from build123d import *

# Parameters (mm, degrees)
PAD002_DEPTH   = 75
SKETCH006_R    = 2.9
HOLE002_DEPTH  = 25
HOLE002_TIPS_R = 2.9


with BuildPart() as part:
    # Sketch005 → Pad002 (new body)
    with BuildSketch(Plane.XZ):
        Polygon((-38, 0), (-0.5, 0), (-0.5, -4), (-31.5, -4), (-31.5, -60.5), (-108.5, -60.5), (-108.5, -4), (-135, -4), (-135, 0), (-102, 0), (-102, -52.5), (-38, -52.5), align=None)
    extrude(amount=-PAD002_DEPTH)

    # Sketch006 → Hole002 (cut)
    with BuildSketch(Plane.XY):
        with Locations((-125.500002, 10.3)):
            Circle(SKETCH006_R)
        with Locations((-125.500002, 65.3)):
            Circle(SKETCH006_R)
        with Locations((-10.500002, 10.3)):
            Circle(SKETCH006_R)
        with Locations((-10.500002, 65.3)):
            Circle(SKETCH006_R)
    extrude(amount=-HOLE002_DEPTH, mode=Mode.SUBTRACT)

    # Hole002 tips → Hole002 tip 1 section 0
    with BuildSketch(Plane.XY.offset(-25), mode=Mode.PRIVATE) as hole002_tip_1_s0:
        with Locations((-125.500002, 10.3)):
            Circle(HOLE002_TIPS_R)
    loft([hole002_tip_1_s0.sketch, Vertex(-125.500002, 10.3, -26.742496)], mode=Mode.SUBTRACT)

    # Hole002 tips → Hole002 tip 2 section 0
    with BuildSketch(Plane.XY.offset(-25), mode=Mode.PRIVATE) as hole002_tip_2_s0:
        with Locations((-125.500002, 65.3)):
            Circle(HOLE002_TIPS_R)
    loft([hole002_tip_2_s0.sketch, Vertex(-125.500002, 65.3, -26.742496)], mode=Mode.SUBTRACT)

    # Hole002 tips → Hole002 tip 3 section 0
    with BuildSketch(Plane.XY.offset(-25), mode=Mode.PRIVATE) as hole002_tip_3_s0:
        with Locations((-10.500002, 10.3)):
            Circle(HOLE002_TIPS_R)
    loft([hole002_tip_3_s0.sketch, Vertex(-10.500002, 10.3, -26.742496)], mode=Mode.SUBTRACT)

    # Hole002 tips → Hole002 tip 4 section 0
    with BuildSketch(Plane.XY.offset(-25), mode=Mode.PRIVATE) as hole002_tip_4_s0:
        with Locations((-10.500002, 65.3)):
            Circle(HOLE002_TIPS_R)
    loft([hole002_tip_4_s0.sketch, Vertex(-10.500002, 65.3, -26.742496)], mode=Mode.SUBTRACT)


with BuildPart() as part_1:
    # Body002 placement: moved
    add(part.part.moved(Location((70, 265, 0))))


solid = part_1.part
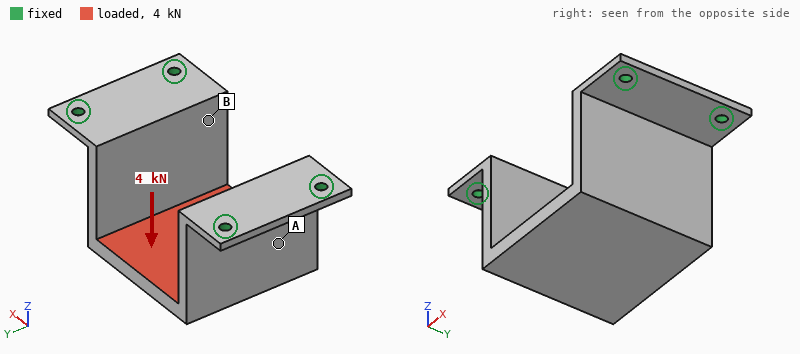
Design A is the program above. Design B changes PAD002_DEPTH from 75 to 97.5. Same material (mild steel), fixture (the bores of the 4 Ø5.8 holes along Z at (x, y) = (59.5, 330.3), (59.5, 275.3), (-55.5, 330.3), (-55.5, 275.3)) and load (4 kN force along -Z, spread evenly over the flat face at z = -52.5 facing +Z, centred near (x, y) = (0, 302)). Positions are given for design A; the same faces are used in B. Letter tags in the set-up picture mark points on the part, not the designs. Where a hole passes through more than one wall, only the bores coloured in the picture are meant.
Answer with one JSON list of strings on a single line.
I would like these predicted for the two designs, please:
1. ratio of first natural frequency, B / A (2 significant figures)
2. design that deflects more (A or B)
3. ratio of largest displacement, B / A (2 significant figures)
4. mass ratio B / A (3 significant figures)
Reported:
["0.93", "B", "1.2", "1.30"]
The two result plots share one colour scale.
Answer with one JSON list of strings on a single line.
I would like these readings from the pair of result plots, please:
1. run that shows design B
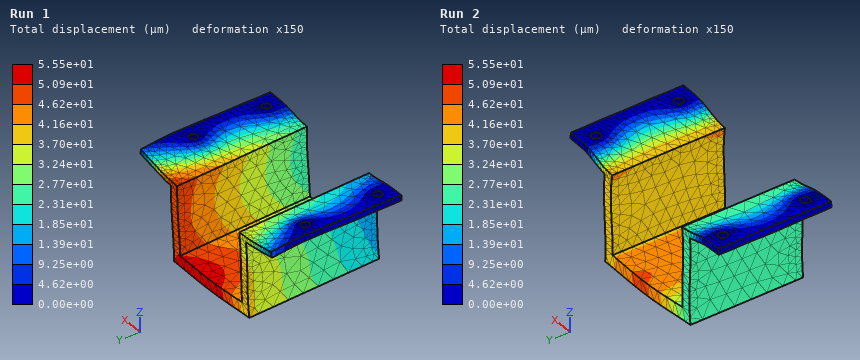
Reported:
["Run 1"]
